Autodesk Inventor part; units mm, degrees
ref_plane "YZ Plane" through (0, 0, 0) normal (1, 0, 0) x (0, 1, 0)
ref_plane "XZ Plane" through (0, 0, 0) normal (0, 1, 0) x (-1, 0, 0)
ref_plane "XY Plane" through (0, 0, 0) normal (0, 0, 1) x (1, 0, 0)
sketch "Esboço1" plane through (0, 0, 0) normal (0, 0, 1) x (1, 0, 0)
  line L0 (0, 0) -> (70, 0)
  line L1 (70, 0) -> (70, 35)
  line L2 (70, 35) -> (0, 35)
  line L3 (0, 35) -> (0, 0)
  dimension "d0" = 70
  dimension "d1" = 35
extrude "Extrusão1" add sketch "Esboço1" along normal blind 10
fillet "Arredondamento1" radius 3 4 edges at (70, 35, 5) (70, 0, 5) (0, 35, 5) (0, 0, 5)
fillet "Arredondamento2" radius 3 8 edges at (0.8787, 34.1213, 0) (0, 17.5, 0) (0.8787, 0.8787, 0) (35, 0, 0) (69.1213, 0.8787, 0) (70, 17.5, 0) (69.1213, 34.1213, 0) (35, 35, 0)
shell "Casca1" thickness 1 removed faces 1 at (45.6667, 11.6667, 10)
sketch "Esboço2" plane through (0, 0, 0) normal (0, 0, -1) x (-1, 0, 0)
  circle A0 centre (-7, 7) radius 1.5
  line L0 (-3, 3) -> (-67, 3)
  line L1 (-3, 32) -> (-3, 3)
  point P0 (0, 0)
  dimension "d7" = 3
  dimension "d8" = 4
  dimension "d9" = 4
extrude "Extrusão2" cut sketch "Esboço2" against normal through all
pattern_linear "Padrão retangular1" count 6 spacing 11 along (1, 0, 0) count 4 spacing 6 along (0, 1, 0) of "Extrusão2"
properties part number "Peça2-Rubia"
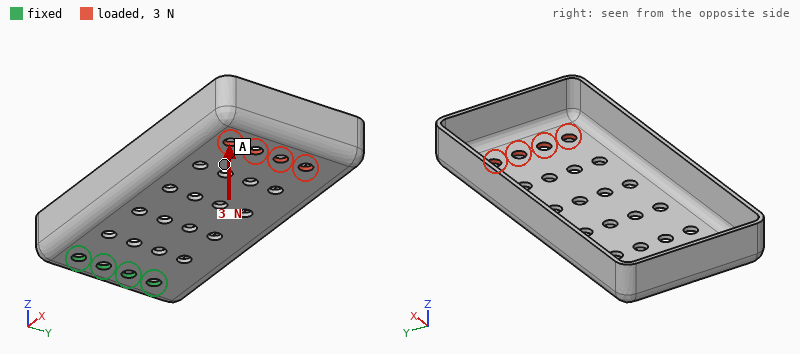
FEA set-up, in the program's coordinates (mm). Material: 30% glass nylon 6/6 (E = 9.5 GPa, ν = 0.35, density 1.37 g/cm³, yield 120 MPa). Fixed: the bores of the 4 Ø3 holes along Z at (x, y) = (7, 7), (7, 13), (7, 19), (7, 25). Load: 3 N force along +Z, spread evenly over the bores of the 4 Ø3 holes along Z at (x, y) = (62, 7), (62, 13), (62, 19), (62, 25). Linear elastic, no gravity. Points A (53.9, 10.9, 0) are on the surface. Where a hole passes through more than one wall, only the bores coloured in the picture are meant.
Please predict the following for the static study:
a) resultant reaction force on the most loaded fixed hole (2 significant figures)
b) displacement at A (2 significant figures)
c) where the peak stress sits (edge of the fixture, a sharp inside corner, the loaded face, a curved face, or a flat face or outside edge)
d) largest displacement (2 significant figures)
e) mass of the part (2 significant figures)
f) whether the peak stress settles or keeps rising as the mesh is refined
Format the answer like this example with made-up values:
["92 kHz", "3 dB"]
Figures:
["7.3 N", "0.52 mm", "edge of the fixture", "0.74 mm", "5.3 g", "keeps rising"]
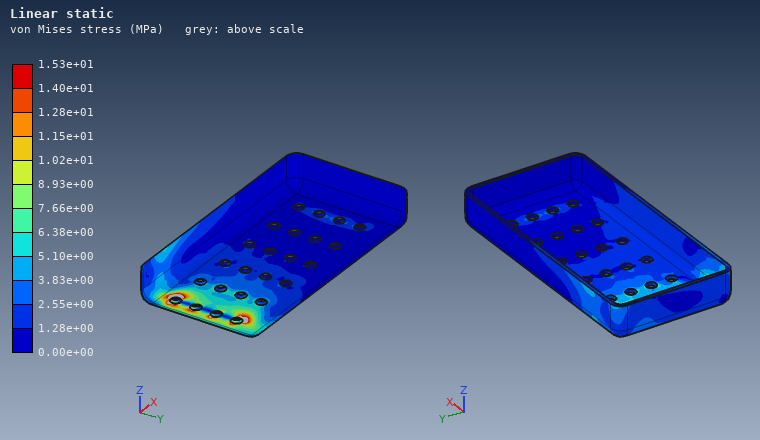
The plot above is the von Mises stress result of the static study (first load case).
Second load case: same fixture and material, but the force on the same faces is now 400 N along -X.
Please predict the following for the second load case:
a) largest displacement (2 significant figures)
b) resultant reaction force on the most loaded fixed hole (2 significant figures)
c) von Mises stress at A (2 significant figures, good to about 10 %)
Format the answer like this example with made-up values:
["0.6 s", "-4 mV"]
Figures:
["0.33 mm", "140 N", "20 MPa"]
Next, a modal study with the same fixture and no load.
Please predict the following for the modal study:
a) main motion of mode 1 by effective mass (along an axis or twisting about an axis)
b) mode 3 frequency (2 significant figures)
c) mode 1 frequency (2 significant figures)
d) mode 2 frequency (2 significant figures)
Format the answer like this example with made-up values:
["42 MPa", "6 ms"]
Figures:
["along Z", "1600 Hz", "230 Hz", "380 Hz"]
